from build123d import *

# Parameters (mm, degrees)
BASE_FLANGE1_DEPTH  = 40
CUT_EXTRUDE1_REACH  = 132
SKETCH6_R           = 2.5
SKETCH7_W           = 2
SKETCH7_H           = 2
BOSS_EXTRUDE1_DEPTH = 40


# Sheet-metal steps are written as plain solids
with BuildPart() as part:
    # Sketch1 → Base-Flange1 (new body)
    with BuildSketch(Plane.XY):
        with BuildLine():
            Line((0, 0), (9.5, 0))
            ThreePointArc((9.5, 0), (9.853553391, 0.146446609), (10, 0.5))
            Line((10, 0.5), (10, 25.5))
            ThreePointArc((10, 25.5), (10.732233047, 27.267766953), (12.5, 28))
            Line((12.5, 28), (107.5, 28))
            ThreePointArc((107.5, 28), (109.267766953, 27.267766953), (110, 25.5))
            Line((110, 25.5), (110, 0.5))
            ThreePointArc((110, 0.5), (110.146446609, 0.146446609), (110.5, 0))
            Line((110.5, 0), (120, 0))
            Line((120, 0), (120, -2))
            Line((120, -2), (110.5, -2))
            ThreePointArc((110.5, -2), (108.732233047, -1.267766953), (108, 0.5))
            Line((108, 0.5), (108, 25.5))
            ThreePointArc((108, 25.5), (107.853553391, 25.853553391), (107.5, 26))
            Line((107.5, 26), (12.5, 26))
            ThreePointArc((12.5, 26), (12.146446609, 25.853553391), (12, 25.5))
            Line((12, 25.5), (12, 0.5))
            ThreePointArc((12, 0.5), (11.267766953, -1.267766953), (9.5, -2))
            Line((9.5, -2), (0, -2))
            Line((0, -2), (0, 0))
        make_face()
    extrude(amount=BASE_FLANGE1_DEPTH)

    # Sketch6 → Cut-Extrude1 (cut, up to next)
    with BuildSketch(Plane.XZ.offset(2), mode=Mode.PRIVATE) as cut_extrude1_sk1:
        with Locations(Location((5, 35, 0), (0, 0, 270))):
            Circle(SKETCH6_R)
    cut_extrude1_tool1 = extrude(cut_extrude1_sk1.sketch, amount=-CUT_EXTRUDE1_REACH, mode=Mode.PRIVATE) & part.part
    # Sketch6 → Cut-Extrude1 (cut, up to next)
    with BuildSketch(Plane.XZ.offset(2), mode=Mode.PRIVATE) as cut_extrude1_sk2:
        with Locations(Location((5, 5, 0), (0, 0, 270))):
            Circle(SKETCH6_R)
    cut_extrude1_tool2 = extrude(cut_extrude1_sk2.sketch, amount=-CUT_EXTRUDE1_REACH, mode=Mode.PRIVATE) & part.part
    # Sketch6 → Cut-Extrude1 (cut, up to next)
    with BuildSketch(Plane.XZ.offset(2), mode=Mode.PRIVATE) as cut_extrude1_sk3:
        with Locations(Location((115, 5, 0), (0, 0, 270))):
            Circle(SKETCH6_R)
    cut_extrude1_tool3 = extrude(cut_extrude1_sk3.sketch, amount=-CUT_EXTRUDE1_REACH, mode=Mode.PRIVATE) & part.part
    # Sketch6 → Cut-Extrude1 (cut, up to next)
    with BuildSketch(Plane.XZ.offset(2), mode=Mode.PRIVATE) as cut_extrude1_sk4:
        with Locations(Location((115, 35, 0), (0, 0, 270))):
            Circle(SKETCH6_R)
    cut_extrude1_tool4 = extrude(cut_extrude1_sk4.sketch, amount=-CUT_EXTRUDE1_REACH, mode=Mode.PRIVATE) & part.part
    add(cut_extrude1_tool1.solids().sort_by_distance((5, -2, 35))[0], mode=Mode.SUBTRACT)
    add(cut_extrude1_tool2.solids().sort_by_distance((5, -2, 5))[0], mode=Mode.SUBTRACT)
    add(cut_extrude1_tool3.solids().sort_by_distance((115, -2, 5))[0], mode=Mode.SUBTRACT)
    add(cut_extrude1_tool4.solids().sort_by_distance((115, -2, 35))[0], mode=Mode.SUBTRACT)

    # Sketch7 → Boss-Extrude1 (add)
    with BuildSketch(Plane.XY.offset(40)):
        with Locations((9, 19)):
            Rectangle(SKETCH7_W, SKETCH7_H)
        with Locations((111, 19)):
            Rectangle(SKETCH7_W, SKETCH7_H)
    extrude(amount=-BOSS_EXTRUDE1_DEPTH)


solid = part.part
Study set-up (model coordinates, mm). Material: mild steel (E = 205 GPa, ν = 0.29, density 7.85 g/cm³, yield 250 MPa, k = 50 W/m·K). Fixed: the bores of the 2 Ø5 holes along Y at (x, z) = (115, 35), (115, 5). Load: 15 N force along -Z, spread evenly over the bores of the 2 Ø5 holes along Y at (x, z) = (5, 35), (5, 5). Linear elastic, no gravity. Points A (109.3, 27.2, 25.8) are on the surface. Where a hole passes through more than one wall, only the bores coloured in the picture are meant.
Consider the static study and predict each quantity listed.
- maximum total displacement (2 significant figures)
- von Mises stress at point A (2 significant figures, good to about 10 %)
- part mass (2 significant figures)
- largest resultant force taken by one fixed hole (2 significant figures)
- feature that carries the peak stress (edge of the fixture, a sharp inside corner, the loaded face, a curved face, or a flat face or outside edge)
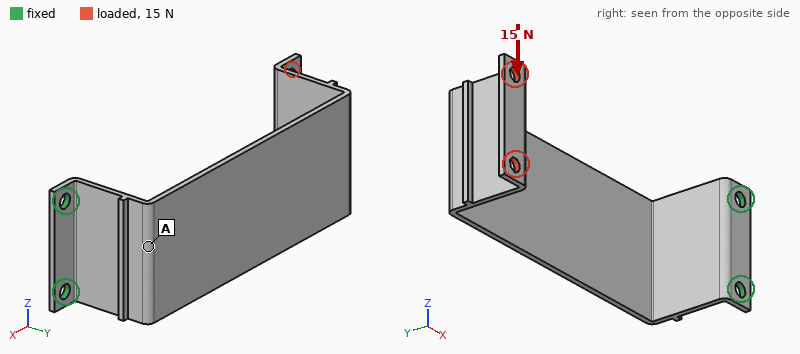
0.51 mm
24 MPa
110 g
52 N
a curved face
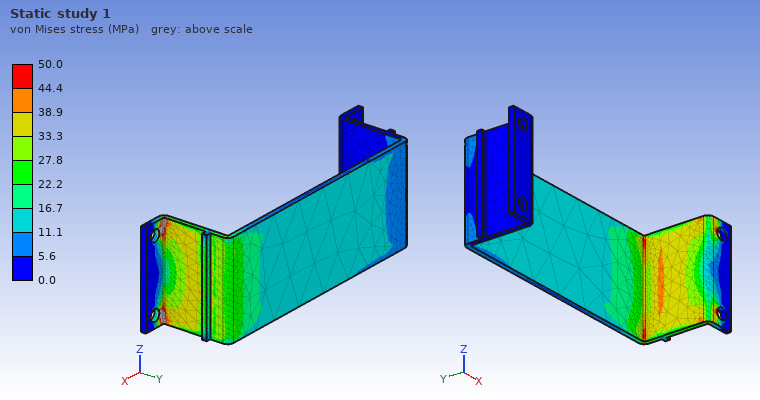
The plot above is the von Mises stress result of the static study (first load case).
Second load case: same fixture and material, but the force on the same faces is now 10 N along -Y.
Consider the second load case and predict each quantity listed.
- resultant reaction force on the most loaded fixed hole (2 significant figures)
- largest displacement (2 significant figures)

5.8 N
1.4 mm
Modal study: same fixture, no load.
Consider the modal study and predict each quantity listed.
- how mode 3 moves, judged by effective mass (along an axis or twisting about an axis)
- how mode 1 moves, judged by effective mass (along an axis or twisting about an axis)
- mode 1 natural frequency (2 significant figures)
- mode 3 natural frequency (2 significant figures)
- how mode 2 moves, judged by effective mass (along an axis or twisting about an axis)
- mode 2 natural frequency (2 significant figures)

along X
along Y
73 Hz
360 Hz
along Z
160 Hz
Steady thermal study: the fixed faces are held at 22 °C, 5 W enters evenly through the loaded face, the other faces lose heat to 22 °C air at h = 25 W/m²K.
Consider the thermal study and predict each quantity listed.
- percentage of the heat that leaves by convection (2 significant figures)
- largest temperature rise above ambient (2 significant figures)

96 %
57 K
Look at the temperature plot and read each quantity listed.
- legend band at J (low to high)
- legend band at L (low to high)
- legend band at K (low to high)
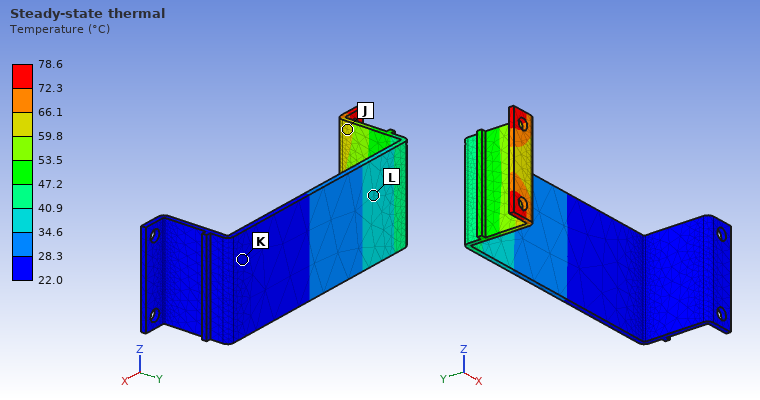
59.8 to 66.1 °C
34.6 to 40.9 °C
22.0 to 28.3 °C
